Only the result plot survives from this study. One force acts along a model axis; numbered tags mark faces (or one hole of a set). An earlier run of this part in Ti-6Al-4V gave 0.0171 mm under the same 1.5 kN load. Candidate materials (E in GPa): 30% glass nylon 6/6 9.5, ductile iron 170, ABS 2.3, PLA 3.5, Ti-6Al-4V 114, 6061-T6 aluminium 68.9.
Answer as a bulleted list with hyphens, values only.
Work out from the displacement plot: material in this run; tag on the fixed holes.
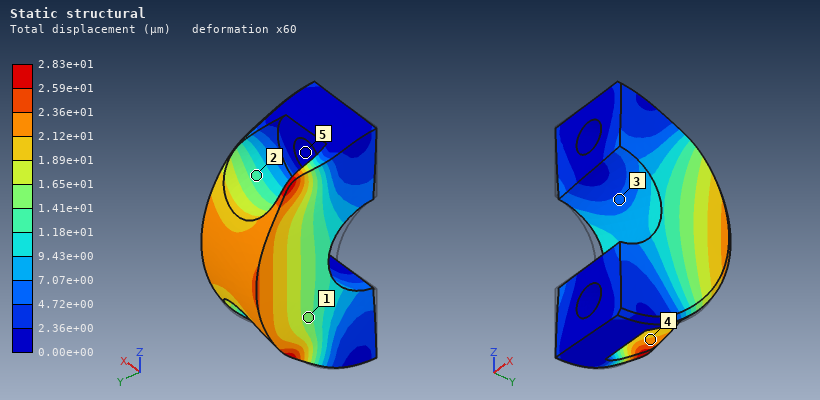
- 6061-T6 aluminium
- 5
